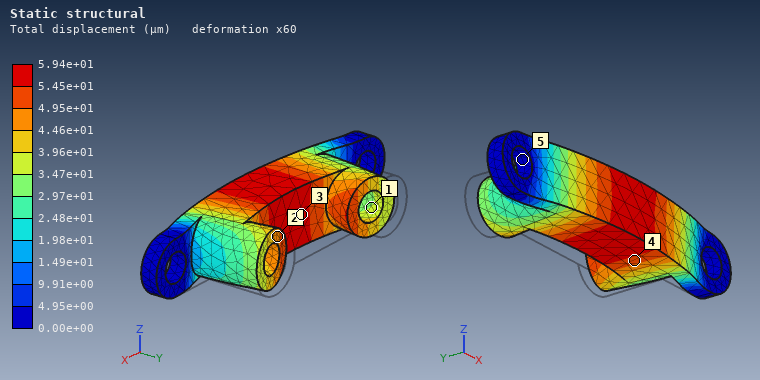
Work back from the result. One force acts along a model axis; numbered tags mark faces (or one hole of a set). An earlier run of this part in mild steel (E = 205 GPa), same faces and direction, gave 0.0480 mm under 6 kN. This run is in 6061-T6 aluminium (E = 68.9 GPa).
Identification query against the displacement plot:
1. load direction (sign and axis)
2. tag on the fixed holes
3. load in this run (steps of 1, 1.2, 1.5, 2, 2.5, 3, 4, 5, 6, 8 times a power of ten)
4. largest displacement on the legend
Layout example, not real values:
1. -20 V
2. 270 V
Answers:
1. -Y
2. 5
3. 2.5 kN
4. 5.94e+01 µm
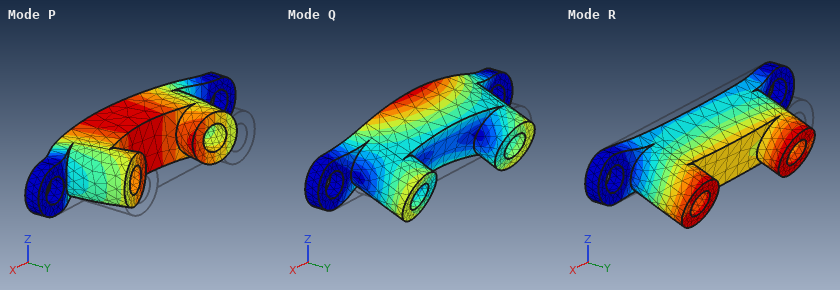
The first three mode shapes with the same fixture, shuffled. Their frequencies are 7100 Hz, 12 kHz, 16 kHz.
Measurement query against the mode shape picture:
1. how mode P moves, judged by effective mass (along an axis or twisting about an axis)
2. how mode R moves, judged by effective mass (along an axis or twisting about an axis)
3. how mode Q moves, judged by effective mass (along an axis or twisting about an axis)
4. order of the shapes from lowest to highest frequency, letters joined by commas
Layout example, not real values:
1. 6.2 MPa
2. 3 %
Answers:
1. along Y
2. along Z
3. along Z
4. R, P, Q
